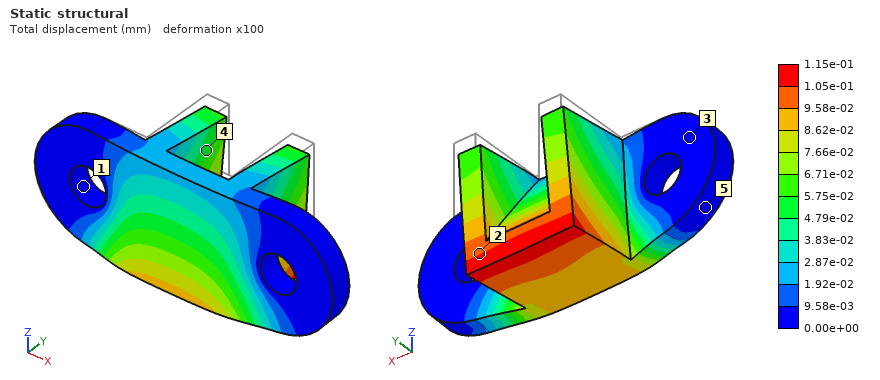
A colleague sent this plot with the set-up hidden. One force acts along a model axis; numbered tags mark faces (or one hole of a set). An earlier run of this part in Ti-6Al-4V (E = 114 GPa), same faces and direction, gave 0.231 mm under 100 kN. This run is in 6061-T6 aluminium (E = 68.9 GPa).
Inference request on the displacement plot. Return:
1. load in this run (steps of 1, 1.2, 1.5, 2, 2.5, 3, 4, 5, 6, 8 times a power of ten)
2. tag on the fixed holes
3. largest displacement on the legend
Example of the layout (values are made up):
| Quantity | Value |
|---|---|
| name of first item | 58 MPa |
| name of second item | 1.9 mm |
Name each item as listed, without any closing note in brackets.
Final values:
| Quantity | Value |
|---|---|
| load in this run | 30 kN |
| tag on the fixed holes | 1 |
| largest displacement on the legend | 1.15e-01 mm |
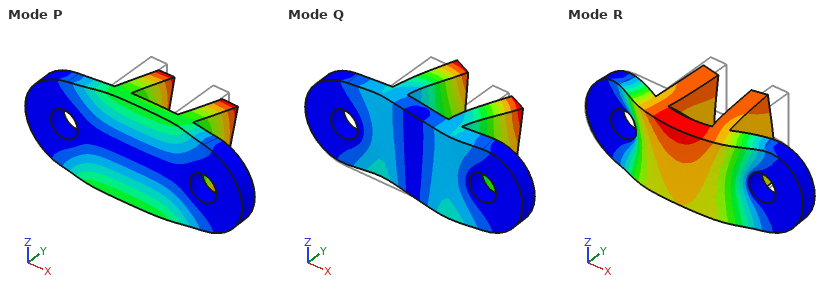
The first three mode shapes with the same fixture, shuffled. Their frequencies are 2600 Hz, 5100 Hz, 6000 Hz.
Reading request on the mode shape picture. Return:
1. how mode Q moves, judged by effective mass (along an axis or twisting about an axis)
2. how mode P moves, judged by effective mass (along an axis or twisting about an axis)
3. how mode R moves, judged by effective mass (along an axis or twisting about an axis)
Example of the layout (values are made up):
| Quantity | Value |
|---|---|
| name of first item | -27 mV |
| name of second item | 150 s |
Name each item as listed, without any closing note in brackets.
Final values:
| Quantity | Value |
|---|---|
| how mode Q moves, judged by effective mass | along X |
| how mode P moves, judged by effective mass | along Z |
| how mode R moves, judged by effective mass | along Y |
